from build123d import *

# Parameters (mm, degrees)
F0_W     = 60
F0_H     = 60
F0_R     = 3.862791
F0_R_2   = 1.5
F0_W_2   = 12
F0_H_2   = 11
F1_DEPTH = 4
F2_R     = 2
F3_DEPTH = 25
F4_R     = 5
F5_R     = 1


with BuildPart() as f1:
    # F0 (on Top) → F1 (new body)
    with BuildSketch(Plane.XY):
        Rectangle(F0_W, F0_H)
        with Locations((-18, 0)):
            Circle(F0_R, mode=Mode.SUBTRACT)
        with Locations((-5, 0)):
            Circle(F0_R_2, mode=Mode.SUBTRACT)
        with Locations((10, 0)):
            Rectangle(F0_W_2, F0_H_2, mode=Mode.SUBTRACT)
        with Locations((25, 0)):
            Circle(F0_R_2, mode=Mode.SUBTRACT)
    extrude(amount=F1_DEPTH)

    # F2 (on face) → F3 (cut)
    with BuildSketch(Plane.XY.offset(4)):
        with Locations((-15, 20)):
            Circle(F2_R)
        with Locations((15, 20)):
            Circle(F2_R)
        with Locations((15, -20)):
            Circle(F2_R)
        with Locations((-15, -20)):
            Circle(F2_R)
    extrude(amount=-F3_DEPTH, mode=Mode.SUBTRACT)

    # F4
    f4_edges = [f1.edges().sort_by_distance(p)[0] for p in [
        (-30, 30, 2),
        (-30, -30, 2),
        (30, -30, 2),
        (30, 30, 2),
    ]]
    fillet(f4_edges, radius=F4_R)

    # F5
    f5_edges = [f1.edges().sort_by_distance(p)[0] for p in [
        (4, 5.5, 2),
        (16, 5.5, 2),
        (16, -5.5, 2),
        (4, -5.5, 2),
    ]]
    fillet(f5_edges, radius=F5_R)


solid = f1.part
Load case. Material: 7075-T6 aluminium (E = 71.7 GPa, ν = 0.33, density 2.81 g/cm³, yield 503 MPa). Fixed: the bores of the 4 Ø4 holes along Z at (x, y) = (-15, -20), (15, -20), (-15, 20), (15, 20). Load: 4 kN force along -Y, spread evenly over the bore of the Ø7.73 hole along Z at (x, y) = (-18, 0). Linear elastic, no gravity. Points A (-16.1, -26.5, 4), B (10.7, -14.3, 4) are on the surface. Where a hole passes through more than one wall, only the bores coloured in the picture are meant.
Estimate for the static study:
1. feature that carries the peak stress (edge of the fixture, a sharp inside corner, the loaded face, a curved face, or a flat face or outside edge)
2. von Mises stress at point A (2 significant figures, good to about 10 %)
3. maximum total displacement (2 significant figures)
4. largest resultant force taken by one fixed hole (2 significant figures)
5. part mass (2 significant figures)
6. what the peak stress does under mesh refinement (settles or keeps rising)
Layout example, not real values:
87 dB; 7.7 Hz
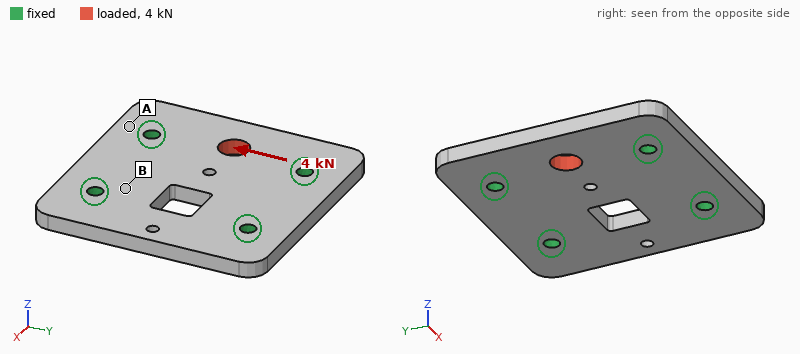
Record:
edge of the fixture; 10 MPa; 11 µm; 1.8 kN; 37 g; keeps rising
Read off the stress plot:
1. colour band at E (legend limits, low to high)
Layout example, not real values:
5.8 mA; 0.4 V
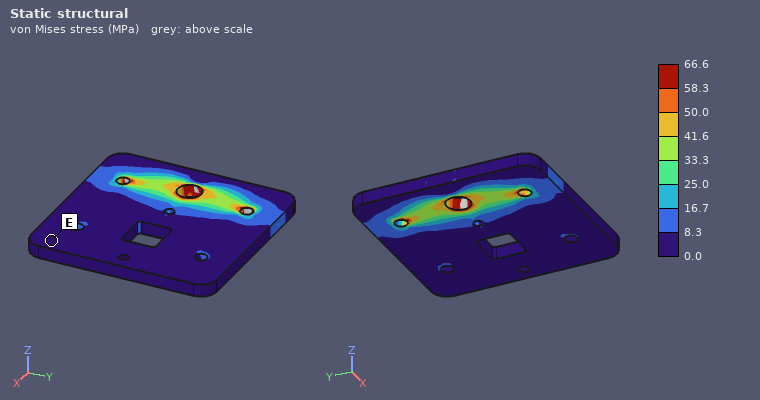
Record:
0.0 to 8.3 MPa
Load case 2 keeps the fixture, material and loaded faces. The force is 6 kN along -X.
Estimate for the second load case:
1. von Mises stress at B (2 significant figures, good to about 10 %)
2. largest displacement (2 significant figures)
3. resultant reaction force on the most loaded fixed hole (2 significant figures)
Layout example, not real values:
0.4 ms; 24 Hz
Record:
28 MPa; 25 µm; 1.9 kN
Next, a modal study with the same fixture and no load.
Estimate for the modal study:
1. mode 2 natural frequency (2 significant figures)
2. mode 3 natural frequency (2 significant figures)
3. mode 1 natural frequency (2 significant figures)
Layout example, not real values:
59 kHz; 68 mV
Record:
9800 Hz; 12 kHz; 9700 Hz
